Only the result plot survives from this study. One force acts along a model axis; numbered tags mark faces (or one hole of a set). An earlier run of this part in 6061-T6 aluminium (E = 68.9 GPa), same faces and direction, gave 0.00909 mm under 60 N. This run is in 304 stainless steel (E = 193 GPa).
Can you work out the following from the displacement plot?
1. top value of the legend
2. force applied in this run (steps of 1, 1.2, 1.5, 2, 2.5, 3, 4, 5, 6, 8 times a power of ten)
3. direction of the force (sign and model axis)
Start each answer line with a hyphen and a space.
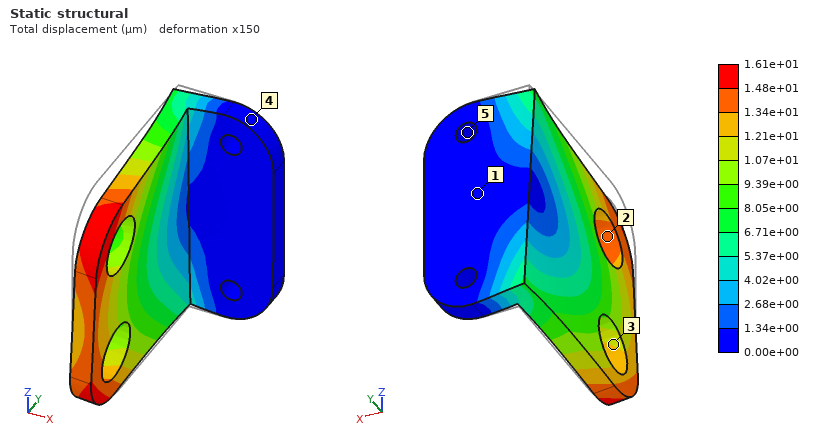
- 1.61e+01 µm
- 300 N
- -Z
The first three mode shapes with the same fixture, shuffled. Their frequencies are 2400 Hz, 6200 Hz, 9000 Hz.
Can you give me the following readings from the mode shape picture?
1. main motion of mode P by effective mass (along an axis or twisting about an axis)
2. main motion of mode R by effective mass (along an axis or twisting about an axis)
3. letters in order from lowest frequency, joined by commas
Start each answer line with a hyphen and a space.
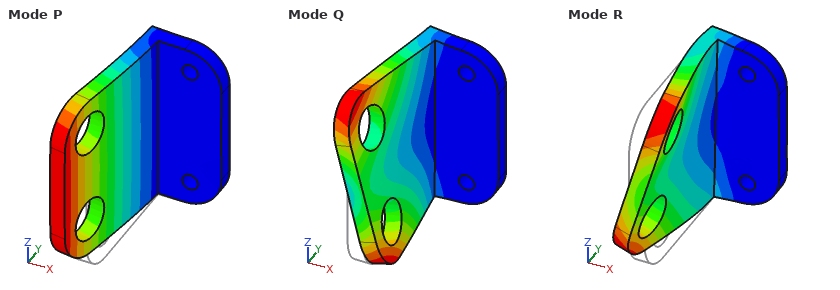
- along X
- along Z
- P, Q, R
